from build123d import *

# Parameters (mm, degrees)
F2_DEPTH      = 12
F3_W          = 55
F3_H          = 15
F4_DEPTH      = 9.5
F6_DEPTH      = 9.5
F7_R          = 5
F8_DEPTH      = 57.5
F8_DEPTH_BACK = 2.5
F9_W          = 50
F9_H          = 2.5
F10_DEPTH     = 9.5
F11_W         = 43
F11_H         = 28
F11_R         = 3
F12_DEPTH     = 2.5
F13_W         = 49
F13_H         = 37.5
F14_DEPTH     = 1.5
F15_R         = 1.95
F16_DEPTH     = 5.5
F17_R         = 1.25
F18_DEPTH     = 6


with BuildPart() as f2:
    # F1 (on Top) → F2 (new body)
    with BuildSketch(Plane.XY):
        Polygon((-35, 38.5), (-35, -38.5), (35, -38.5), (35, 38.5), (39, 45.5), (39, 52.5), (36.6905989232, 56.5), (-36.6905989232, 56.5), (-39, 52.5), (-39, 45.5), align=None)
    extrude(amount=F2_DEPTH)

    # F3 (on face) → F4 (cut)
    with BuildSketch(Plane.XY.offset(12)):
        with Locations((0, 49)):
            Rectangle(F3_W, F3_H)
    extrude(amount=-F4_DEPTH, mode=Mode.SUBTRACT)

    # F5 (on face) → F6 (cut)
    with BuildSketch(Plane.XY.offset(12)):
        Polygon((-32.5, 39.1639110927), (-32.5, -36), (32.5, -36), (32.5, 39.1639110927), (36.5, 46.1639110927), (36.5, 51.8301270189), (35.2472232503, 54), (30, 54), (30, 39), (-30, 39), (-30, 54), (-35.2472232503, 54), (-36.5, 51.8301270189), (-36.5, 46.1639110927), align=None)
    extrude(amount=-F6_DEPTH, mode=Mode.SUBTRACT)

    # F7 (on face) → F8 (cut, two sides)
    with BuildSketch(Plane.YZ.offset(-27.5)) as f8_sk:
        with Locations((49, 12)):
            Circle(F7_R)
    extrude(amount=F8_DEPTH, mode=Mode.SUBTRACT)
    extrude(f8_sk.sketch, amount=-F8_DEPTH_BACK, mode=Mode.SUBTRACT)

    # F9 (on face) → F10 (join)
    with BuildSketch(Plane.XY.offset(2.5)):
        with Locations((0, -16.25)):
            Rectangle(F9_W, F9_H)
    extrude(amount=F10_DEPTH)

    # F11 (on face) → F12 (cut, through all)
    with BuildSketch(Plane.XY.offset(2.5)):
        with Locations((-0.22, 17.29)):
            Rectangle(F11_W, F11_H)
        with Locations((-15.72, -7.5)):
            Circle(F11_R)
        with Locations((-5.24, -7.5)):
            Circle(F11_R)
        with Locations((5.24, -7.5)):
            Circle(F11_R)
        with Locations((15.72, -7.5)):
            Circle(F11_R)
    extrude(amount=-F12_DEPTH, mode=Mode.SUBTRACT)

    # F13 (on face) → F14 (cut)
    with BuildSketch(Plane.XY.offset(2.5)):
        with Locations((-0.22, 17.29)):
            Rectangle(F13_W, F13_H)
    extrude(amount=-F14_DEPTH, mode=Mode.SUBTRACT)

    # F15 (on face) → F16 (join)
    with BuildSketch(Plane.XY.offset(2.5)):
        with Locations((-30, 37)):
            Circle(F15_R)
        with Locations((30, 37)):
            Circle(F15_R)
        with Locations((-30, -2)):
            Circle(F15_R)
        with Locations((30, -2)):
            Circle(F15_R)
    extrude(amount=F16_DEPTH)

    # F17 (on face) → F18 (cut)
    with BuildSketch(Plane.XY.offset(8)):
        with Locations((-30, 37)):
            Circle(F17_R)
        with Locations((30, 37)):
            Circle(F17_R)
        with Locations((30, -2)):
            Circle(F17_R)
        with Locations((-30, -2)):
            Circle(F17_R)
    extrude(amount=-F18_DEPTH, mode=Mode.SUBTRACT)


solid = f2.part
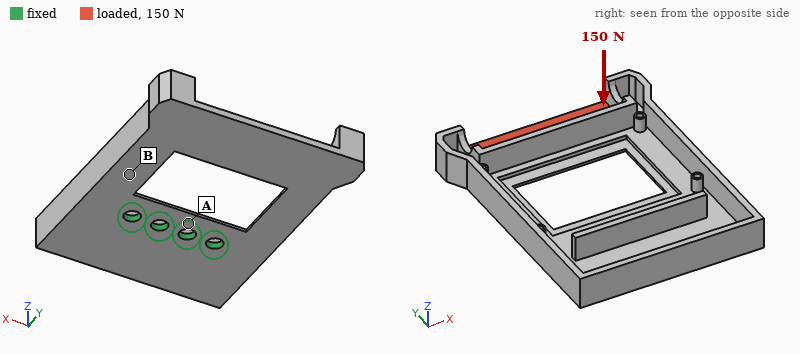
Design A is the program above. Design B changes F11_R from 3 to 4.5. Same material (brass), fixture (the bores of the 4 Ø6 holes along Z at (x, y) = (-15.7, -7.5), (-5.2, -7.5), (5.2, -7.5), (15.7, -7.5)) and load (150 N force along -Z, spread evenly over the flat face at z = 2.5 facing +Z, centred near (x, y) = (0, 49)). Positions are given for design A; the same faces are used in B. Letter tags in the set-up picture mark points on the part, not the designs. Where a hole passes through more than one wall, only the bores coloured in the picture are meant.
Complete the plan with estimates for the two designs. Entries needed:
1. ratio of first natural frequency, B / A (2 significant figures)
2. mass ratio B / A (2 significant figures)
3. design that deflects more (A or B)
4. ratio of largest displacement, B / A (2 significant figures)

1.1
0.98
A
0.80
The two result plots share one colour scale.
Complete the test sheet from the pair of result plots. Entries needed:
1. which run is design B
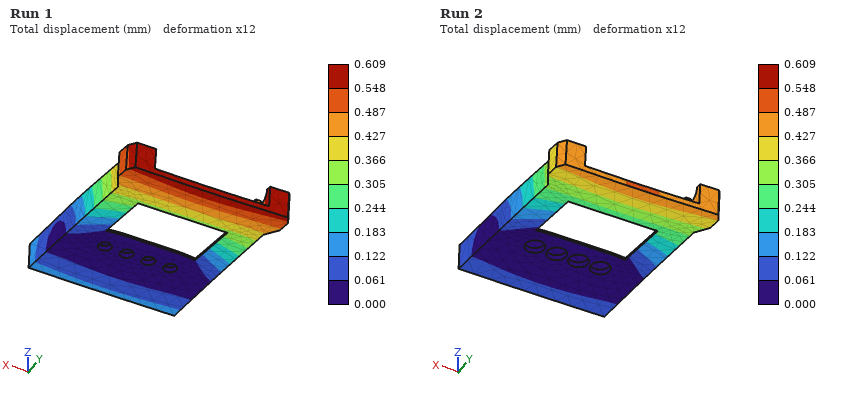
Run 2
